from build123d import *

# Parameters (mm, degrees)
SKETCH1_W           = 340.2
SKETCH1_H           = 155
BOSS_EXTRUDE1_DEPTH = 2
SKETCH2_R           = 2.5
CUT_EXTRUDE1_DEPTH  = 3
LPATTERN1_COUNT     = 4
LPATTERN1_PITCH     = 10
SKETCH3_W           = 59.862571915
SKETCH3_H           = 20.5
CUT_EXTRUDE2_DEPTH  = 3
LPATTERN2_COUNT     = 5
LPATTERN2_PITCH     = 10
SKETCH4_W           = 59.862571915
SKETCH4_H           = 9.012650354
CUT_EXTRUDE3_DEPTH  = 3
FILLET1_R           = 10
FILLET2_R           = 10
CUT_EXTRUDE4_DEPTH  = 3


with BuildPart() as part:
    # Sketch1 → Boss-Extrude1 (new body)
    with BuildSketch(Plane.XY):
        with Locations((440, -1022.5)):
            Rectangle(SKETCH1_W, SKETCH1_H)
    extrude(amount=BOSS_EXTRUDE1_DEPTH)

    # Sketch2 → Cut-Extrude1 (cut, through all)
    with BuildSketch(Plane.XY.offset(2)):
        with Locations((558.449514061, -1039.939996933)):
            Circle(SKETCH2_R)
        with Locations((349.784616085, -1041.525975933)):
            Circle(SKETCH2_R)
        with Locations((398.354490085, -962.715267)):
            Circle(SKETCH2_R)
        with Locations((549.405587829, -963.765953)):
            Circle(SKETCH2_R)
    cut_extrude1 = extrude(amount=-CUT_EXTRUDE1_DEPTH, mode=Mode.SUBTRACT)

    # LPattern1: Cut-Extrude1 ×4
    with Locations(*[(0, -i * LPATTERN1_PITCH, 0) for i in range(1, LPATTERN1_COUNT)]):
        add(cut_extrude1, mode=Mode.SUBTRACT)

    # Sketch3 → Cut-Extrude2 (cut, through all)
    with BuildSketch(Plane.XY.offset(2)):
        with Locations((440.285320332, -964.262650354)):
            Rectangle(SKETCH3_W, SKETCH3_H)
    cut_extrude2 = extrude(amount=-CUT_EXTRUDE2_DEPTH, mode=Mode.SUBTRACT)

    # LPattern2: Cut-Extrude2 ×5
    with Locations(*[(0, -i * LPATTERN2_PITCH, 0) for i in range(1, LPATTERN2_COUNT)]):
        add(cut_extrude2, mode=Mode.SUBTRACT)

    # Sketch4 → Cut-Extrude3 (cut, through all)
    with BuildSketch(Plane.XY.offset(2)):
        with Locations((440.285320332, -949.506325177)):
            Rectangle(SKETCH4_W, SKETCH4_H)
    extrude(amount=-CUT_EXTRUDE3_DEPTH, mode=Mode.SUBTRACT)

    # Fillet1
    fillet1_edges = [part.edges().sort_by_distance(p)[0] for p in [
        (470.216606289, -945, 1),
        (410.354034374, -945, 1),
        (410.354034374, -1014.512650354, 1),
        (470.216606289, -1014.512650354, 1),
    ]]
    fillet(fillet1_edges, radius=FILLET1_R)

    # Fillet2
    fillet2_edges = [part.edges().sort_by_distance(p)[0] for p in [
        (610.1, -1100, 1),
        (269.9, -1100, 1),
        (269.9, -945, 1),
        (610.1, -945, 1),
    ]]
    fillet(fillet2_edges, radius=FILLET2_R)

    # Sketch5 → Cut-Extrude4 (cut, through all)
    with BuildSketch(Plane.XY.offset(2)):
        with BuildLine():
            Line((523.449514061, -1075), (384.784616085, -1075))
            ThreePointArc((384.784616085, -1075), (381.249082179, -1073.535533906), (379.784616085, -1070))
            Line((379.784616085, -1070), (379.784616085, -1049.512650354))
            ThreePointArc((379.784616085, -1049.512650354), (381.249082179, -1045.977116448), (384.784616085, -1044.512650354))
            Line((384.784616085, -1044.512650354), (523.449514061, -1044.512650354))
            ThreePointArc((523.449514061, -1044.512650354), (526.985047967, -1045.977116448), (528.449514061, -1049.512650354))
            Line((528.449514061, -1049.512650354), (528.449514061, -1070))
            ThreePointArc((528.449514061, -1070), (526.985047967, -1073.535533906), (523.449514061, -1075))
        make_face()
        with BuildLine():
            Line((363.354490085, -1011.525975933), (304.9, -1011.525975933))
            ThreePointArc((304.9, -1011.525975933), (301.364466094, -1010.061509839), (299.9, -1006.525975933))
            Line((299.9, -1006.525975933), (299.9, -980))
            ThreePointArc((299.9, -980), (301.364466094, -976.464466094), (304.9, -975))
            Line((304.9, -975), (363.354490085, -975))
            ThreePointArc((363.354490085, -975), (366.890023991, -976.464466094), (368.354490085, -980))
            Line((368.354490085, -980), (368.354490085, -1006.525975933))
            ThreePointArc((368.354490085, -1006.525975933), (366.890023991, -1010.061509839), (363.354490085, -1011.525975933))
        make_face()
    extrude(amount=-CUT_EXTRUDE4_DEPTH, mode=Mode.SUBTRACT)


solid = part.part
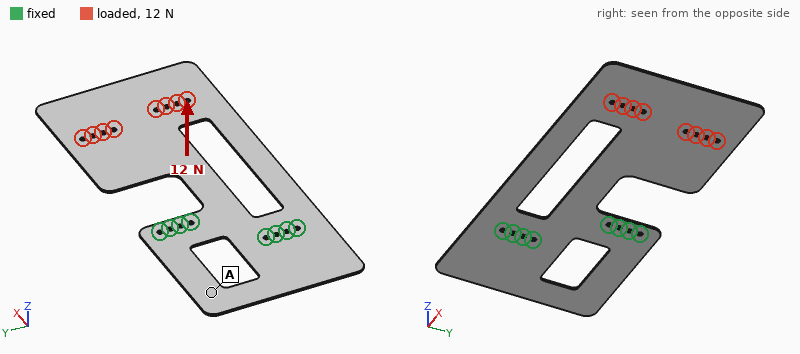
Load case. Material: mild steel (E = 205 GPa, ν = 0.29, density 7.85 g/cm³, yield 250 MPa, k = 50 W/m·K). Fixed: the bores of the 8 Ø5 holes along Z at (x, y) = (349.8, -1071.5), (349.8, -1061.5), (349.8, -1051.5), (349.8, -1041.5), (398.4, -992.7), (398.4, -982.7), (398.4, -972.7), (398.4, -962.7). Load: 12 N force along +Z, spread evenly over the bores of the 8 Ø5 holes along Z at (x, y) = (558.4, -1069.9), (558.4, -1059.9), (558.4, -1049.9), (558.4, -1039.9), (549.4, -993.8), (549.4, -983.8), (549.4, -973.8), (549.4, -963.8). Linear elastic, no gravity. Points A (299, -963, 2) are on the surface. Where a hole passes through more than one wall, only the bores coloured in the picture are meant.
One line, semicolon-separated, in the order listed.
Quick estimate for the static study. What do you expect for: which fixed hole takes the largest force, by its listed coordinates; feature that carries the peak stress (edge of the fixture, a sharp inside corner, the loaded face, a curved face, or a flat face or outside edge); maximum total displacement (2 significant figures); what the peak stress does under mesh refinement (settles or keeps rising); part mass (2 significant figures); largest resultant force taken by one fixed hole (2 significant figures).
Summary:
(398.4, -992.7); edge of the fixture; 4.0 mm; keeps rising; 650 g; 45 N
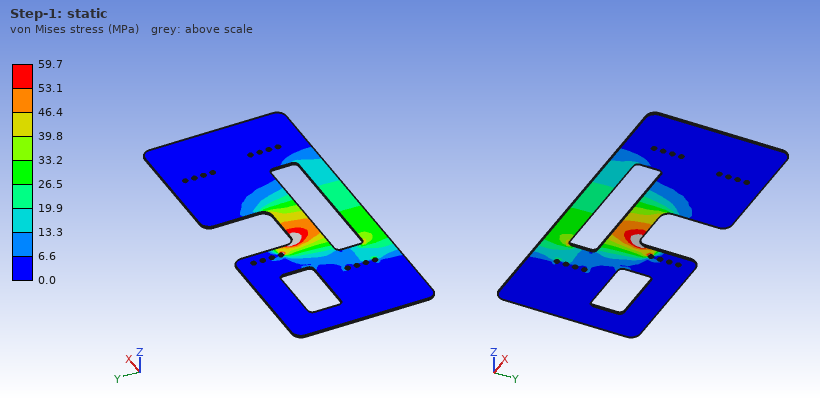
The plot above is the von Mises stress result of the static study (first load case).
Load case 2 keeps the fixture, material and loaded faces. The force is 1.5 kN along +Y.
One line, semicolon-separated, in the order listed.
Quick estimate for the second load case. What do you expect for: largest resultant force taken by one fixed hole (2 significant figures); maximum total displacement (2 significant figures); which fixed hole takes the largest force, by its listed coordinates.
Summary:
2.8 kN; 0.47 mm; (349.8, -1071.5)
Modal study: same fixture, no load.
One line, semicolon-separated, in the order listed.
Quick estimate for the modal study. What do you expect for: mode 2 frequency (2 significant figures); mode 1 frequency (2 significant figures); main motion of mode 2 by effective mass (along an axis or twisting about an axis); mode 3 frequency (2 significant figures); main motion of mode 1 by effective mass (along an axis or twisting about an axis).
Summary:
63 Hz; 20 Hz; twisting about X; 160 Hz; along Z
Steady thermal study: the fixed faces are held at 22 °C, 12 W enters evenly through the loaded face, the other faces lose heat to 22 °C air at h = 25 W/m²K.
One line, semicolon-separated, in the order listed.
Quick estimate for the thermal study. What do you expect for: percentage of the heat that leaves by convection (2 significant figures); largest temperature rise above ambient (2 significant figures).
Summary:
99 %; 25 K
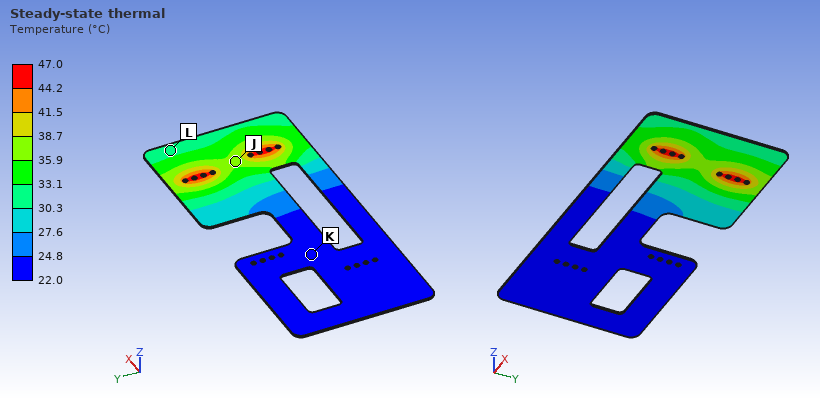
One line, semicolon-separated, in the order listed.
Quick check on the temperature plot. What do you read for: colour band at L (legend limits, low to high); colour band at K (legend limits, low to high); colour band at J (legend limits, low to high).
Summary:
30.3 to 33.1 °C; 22.0 to 24.8 °C; 35.9 to 38.7 °C
